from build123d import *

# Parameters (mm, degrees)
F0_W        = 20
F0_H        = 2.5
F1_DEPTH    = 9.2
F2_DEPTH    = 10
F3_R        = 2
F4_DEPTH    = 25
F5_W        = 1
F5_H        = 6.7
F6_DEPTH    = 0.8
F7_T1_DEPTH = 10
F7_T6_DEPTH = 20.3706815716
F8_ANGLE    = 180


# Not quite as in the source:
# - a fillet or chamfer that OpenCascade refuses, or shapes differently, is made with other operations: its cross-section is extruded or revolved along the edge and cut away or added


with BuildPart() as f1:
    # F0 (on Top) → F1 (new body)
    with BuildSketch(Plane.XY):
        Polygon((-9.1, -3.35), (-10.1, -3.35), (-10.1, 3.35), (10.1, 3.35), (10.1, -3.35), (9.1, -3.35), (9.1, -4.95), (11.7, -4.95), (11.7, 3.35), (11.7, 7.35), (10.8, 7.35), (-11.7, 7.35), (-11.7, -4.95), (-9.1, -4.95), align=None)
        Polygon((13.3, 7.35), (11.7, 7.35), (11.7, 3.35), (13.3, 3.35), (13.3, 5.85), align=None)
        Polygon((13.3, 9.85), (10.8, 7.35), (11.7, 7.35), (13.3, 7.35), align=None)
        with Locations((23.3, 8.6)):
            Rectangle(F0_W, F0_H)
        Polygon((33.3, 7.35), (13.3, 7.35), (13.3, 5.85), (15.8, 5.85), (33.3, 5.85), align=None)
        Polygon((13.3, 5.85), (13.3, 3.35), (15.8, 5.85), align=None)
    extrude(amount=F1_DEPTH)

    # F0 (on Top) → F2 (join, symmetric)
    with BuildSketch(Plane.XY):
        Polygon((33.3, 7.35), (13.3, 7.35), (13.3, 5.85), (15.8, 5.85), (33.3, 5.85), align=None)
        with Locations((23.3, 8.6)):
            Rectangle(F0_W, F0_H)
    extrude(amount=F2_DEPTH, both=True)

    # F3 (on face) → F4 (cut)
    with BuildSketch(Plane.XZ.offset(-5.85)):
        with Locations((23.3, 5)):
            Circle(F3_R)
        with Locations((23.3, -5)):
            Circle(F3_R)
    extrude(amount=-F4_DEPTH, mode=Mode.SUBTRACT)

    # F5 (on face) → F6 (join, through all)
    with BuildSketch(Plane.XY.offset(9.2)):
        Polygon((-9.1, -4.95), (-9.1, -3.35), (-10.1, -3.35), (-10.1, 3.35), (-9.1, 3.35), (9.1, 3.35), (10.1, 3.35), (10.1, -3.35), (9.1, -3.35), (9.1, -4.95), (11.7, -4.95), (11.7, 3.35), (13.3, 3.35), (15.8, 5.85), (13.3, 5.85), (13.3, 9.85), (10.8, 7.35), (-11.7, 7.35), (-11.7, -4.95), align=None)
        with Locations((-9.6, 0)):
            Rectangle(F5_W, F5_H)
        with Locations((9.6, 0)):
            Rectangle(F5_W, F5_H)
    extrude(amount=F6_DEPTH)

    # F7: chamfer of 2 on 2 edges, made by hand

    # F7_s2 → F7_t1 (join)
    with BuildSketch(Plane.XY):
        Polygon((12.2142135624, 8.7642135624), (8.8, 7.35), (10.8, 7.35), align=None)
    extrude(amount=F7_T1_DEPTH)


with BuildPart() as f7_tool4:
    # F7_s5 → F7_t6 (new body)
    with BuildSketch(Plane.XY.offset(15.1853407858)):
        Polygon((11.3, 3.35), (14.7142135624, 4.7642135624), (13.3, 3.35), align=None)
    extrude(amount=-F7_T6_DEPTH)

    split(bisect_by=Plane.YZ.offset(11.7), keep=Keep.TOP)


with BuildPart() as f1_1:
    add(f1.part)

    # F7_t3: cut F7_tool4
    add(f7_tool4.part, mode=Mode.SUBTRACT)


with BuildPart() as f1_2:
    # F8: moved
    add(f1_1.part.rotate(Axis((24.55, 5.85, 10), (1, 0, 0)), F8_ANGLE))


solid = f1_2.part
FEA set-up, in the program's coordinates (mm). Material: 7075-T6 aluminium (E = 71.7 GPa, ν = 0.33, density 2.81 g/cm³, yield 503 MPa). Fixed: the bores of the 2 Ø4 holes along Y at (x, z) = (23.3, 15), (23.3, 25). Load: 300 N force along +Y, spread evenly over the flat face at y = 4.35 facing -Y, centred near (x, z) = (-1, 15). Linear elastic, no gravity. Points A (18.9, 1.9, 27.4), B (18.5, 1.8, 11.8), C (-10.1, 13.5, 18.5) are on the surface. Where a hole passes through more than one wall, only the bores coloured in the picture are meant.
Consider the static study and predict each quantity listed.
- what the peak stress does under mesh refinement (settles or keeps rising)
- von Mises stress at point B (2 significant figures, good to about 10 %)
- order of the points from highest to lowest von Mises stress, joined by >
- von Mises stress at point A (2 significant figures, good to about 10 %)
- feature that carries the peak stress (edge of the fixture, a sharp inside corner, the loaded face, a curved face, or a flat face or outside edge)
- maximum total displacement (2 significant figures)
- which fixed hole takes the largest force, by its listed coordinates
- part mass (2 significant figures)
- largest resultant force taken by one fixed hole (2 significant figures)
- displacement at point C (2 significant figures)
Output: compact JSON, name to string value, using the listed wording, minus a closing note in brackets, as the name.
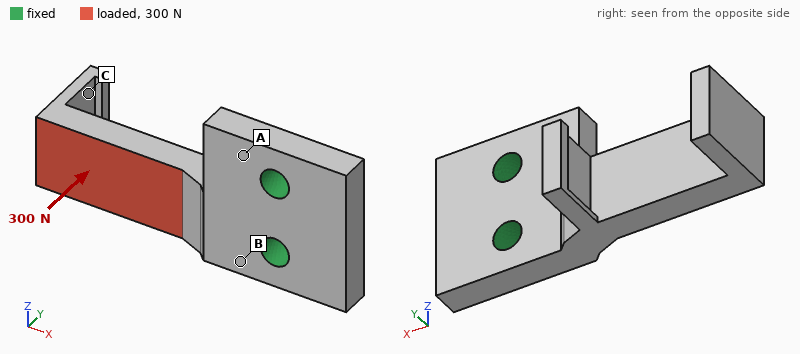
{"what the peak stress does under mesh refinement": "keeps rising", "von Mises stress at point B": "160 MPa", "order of the points from highest to lowest von Mises stress, joined by >": "B > A > C", "von Mises stress at point A": "55 MPa", "feature that carries the peak stress": "edge of the fixture", "maximum total displacement": "0.49 mm", "which fixed hole takes the largest force, by its listed coordinates": "(23.3, 15)", "part mass": "8.1 g", "largest resultant force taken by one fixed hole": "250 N", "displacement at point C": "0.43 mm"}
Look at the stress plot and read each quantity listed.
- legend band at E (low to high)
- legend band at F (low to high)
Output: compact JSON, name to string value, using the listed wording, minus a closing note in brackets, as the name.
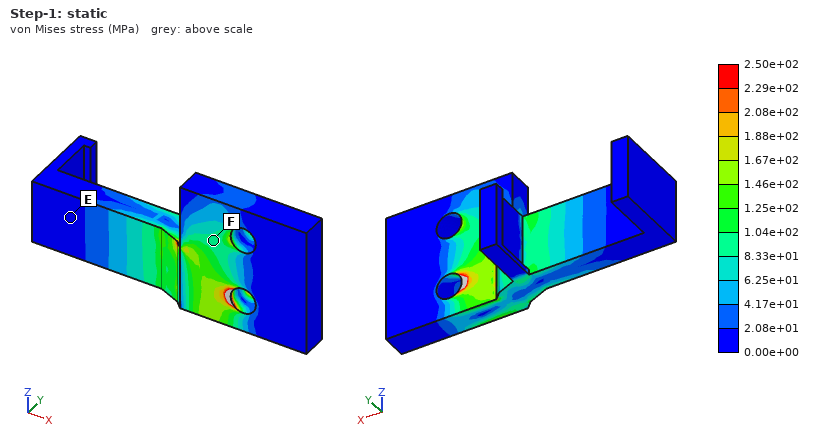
{"legend band at E": "0.00e+00 to 2.08e+01 MPa", "legend band at F": "8.33e+01 to 1.04e+02 MPa"}
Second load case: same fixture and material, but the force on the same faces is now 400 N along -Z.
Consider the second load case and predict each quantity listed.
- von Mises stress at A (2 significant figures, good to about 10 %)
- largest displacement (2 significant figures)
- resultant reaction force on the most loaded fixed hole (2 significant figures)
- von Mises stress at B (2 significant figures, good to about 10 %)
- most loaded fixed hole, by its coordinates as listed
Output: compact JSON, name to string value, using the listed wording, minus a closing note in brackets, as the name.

{"von Mises stress at A": "11 MPa", "largest displacement": "0.11 mm", "resultant reaction force on the most loaded fixed hole": "880 N", "von Mises stress at B": "32 MPa", "most loaded fixed hole, by its coordinates as listed": "(23.3, 25)"}
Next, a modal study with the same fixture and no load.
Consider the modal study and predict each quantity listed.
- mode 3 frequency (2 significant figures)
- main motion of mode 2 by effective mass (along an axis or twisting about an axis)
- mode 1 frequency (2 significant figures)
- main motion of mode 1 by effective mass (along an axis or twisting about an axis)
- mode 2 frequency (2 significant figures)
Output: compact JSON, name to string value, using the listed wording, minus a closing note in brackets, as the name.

{"mode 3 frequency": "11 kHz", "main motion of mode 2 by effective mass": "along Z", "mode 1 frequency": "2600 Hz", "main motion of mode 1 by effective mass": "along Y", "mode 2 frequency": "6500 Hz"}
